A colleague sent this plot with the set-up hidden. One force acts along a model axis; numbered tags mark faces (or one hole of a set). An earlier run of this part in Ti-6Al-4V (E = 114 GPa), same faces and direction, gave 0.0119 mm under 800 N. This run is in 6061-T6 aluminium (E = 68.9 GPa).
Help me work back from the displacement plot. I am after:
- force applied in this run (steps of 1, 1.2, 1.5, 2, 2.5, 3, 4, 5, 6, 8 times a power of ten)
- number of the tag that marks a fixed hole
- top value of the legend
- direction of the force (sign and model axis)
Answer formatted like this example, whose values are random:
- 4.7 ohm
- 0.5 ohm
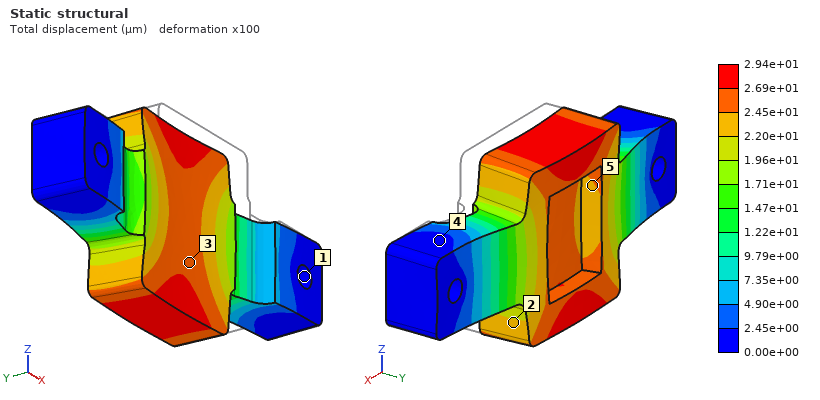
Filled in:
- 1.2 kN
- 1
- 2.94e+01 µm
- +Y
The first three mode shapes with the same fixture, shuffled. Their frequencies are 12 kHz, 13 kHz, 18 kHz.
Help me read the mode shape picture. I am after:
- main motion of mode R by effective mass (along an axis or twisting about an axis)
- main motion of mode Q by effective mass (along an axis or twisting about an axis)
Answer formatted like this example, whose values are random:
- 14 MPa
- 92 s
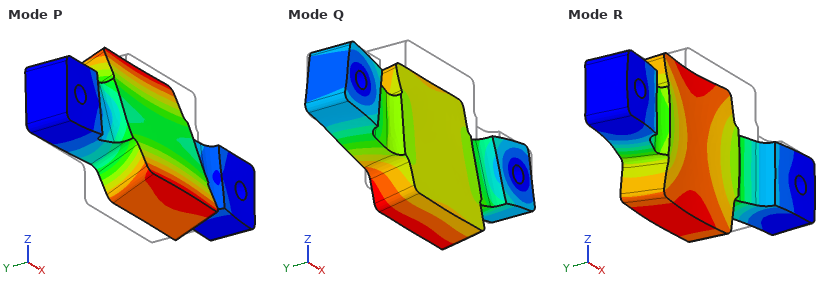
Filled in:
- along Y
- along Z
